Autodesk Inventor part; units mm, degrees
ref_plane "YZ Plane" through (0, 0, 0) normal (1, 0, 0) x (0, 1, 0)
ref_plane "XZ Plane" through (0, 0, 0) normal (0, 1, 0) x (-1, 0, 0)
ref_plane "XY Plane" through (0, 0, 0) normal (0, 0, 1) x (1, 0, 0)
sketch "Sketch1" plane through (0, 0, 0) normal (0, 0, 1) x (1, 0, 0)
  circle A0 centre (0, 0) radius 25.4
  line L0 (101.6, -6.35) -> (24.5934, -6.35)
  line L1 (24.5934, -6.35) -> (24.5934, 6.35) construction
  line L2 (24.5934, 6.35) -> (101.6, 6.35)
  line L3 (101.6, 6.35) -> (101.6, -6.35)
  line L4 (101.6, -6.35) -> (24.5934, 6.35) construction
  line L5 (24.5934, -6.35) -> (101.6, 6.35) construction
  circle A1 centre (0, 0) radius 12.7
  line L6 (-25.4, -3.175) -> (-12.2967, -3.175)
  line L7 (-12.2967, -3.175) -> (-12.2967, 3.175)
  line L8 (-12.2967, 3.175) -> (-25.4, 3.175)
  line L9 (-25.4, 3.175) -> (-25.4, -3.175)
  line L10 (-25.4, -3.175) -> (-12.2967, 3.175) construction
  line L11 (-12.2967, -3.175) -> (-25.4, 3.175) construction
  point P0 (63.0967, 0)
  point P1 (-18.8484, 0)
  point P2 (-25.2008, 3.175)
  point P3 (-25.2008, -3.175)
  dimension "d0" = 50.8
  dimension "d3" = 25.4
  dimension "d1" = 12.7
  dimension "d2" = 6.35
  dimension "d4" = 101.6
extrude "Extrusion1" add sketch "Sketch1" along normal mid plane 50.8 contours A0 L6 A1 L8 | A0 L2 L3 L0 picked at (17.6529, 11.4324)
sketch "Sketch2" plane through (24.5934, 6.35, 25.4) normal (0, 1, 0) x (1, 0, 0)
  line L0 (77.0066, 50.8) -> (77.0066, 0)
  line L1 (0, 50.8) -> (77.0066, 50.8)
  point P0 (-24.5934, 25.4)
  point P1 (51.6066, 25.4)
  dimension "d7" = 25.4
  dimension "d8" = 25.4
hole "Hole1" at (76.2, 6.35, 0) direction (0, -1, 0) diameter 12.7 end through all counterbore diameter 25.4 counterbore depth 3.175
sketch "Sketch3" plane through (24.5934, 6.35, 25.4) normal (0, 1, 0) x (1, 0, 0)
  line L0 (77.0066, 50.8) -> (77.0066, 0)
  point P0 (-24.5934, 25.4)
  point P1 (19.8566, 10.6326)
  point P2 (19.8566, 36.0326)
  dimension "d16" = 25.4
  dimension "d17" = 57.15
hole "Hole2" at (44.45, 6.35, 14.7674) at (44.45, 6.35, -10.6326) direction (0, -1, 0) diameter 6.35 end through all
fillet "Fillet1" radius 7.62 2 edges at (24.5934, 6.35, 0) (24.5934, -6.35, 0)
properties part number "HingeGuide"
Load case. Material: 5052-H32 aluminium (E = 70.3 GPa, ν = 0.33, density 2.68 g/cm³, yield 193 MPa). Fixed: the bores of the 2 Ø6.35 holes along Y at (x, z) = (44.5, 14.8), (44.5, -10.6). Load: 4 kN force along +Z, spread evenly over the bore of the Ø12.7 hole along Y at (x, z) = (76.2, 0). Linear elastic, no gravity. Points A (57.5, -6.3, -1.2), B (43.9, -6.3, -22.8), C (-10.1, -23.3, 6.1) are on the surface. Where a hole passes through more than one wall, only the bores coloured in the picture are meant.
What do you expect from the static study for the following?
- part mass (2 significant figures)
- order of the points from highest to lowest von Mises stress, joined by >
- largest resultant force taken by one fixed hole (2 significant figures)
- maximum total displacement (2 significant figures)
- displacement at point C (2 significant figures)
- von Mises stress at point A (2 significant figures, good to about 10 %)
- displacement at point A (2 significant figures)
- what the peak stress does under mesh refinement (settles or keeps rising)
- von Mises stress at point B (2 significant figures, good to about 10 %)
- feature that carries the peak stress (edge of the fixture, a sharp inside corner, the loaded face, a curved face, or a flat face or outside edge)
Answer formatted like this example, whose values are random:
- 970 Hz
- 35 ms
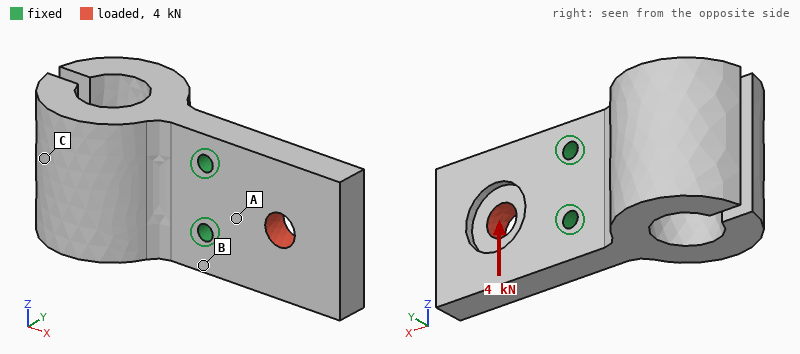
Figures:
- 320 g
- A > B > C
- 4.7 kN
- 30 µm
- 5.7 µm
- 23 MPa
- 5.7 µm
- keeps rising
- 10 MPa
- edge of the fixture
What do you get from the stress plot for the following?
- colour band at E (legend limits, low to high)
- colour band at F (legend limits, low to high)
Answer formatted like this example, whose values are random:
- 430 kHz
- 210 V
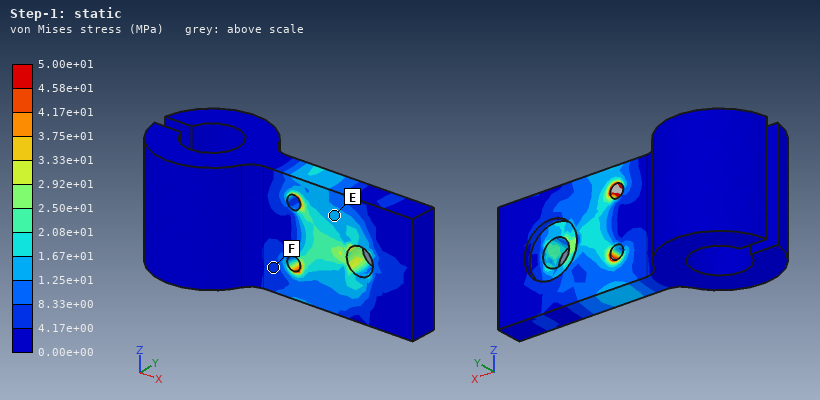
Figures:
- 1.25e+01 to 1.67e+01 MPa
- 4.17e+00 to 8.33e+00 MPa
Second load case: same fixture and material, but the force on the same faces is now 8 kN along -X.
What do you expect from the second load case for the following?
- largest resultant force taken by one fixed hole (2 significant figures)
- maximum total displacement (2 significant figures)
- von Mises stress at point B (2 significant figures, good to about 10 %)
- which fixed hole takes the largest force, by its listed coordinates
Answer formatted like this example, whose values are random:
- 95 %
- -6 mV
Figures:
- 4.6 kN
- 29 µm
- 10 MPa
- (44.5, -10.6)
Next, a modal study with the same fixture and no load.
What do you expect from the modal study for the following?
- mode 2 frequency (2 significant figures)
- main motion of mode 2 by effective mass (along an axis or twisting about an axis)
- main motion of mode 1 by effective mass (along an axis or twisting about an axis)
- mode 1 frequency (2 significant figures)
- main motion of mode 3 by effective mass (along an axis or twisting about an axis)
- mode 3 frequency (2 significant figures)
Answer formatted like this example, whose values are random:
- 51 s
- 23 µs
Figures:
- 3100 Hz
- along Y
- along Y
- 1500 Hz
- along Z
- 3900 Hz
